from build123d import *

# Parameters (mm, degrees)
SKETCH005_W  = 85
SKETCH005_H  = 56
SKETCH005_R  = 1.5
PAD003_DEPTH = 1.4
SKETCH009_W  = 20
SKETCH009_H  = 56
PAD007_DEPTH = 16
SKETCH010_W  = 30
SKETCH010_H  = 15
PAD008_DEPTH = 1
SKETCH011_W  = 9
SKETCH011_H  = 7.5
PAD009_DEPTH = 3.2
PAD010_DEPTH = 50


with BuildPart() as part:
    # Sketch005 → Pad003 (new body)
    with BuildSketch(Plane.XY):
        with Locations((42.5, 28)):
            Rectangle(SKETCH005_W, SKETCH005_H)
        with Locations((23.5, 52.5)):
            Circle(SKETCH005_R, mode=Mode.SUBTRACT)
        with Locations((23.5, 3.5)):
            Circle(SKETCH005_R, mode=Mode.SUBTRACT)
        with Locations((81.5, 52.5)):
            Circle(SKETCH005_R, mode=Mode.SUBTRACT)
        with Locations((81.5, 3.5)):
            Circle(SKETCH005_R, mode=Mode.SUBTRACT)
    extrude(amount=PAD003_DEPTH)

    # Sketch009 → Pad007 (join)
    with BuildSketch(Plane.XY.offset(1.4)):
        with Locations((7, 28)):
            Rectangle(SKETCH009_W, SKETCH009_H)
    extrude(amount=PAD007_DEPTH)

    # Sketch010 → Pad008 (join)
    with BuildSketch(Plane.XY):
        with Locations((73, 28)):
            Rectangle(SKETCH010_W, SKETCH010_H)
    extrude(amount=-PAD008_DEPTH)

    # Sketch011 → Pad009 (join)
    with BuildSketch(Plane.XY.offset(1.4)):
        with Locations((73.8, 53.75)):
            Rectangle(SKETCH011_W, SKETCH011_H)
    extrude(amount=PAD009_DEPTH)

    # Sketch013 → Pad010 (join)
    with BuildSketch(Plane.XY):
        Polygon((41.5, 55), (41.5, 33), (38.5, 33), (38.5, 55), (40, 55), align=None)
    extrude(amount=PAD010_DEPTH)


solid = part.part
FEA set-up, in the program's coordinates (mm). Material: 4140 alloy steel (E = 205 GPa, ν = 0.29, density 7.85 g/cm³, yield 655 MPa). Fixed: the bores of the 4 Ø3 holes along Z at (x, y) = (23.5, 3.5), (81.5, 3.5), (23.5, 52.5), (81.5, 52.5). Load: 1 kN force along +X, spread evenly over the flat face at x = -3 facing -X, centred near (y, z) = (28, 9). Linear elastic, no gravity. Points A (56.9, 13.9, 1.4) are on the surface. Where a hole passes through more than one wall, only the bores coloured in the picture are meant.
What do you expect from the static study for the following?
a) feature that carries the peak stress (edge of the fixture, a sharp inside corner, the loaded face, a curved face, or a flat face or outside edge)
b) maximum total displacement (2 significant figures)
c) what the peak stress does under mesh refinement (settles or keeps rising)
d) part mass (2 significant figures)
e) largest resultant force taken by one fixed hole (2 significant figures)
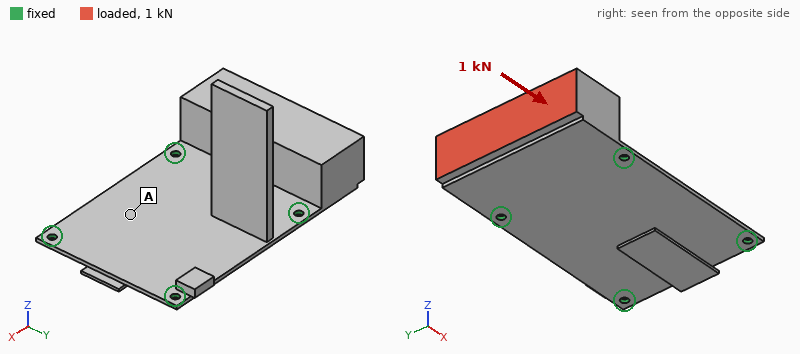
edge of the fixture
0.79 mm
keeps rising
220 g
420 N
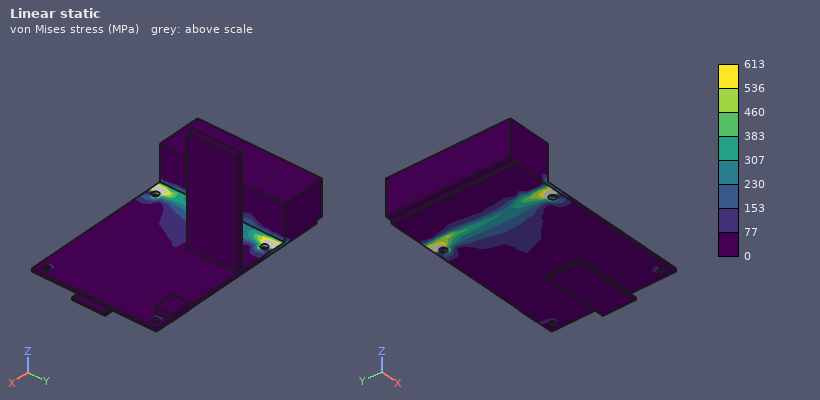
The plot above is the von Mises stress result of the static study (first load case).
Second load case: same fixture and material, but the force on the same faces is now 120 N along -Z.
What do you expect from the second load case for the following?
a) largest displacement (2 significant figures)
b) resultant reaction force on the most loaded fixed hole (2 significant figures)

0.25 mm
67 N
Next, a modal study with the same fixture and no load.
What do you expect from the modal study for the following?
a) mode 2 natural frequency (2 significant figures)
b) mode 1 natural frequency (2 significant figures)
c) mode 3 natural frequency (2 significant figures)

560 Hz
420 Hz
860 Hz
